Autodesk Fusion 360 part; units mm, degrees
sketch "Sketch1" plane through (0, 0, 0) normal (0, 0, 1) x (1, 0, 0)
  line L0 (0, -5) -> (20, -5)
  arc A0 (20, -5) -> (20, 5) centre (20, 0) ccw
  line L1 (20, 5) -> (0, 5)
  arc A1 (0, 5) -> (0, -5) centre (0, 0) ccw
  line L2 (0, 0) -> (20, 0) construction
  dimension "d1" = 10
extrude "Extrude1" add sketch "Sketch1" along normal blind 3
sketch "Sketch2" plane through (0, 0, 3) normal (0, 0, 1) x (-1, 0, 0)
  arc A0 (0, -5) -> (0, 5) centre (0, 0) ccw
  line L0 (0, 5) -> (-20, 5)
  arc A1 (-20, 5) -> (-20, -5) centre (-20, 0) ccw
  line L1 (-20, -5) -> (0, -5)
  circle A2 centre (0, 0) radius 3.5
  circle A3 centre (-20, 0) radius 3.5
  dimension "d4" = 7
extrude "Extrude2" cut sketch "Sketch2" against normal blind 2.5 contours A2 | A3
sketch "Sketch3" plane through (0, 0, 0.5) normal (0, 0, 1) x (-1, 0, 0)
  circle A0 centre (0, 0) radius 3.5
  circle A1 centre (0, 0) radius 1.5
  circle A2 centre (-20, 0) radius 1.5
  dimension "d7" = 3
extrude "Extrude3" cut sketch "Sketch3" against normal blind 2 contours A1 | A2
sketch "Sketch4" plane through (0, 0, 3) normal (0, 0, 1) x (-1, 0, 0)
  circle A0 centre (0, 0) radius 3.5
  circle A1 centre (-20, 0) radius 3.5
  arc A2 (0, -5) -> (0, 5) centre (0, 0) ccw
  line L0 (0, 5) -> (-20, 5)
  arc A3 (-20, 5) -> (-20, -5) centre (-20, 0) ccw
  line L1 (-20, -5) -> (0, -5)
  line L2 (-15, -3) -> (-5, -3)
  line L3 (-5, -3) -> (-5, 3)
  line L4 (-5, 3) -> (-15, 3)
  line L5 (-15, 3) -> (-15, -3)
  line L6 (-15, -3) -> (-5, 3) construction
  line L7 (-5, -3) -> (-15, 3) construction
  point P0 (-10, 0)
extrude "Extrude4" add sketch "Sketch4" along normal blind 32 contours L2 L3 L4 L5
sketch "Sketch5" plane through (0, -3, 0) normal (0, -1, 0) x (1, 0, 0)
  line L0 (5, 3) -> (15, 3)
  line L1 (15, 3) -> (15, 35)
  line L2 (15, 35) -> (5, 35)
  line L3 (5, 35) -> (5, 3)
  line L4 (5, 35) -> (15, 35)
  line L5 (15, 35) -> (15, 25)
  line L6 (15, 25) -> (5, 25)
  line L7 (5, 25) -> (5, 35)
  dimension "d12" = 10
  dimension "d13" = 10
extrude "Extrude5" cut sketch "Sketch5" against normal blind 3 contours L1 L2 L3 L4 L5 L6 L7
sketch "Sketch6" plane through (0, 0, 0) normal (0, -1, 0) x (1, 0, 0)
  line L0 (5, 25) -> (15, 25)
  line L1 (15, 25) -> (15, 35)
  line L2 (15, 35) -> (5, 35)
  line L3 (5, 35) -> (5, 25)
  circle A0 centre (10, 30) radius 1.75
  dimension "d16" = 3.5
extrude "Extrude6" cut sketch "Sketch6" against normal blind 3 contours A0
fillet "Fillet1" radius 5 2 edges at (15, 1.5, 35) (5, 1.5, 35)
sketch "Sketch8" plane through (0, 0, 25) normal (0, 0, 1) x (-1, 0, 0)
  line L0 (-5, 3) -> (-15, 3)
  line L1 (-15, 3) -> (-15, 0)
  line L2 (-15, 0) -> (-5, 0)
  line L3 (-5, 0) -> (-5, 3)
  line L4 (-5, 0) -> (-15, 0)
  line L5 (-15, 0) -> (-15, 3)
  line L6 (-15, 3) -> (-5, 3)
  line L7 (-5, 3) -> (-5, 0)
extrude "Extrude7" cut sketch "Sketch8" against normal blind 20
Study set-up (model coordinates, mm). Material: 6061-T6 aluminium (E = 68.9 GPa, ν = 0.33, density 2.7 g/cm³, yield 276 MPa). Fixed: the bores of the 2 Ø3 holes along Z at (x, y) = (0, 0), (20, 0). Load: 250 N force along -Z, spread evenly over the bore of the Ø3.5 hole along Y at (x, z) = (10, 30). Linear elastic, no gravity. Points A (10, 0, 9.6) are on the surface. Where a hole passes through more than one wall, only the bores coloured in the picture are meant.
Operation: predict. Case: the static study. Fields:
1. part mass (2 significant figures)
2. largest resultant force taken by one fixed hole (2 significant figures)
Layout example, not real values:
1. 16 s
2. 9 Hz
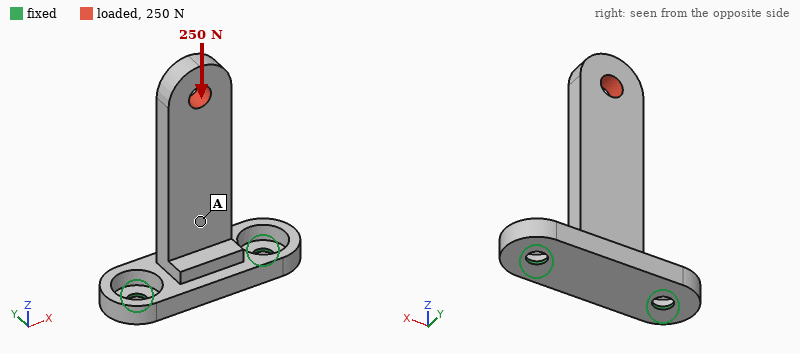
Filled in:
1. 4.3 g
2. 180 N
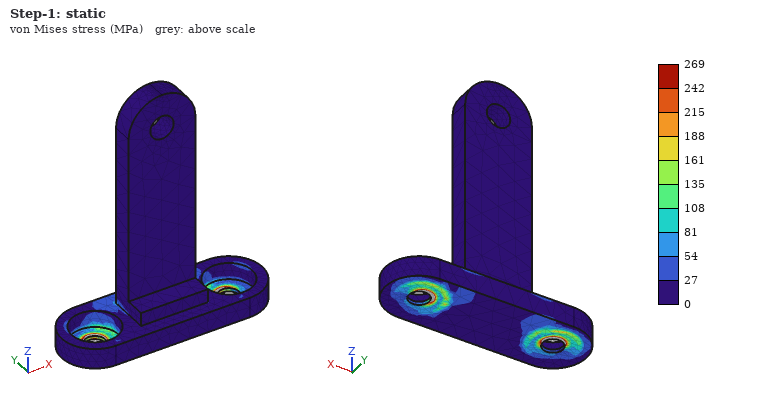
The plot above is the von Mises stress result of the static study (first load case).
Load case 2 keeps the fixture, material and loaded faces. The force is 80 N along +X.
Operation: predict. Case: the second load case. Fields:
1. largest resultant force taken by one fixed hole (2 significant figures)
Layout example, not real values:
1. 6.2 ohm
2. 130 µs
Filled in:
1. 130 N
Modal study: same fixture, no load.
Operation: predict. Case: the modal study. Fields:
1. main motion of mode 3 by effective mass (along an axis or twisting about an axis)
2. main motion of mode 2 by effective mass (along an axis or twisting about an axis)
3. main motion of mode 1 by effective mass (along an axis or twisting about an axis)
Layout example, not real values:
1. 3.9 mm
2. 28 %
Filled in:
1. along Z
2. along X
3. along Y
